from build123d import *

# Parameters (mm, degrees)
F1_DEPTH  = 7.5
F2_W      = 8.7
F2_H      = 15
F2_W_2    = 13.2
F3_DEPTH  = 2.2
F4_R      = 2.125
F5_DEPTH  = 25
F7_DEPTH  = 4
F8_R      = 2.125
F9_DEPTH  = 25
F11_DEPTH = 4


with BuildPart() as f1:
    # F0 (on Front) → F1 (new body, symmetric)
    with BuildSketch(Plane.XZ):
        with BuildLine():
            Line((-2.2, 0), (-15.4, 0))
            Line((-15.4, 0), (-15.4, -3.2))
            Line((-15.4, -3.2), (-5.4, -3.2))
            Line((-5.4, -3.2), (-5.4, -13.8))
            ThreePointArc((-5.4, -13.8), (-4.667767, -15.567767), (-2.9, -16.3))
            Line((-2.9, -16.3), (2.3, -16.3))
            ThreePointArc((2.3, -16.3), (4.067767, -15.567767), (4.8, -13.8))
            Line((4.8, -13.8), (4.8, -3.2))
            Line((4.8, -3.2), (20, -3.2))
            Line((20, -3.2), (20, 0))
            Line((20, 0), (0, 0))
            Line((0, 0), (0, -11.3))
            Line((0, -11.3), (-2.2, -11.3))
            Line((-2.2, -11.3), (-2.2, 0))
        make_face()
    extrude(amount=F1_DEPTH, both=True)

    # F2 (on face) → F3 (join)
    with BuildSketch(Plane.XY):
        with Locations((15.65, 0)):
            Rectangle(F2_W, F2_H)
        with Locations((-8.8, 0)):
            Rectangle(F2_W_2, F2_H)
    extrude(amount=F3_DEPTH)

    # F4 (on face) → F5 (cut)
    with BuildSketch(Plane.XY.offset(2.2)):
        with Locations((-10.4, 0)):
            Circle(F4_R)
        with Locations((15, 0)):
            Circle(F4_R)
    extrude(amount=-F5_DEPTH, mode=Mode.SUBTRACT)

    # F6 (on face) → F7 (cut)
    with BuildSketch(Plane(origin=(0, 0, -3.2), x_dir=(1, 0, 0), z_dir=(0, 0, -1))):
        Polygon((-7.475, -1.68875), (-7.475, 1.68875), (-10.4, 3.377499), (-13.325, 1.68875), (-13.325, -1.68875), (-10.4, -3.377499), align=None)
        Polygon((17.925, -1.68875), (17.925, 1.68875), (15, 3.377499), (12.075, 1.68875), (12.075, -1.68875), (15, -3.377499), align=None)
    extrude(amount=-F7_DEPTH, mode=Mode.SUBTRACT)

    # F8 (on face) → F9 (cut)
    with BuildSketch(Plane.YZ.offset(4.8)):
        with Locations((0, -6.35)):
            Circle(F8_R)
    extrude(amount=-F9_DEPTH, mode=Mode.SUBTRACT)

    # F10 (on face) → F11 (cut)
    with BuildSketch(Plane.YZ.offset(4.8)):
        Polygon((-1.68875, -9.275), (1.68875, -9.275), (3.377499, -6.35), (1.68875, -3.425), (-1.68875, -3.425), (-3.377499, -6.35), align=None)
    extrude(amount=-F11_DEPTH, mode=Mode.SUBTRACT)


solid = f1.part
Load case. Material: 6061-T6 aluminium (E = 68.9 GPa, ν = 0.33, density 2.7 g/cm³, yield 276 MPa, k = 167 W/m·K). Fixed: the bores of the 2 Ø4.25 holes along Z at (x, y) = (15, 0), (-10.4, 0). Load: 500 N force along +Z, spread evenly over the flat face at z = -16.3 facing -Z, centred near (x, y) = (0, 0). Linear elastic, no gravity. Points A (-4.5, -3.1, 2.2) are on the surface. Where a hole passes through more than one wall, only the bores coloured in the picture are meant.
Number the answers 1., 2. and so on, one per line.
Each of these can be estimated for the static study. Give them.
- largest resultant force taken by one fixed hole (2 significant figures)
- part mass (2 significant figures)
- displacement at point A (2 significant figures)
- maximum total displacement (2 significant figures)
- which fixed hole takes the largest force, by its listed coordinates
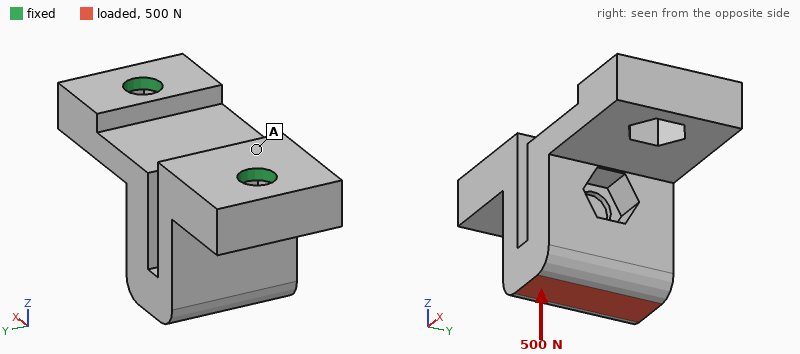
1. 330 N
2. 9.6 g
3. 5.8 µm
4. 15 µm
5. (-10.4, 0)
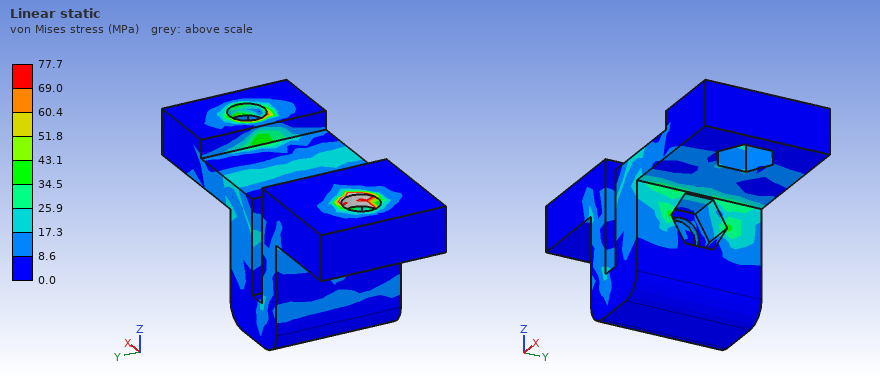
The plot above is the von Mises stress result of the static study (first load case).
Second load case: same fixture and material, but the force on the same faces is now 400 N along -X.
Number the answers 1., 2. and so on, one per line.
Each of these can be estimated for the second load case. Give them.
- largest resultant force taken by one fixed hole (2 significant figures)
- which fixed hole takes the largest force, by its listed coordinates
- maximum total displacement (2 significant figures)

1. 410 N
2. (15, 0)
3. 35 µm
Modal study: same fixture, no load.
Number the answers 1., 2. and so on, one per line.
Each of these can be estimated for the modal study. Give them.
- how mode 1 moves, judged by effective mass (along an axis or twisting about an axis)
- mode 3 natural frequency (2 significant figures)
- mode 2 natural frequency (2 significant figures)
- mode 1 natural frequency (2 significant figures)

1. along Y
2. 17 kHz
3. 12 kHz
4. 5800 Hz
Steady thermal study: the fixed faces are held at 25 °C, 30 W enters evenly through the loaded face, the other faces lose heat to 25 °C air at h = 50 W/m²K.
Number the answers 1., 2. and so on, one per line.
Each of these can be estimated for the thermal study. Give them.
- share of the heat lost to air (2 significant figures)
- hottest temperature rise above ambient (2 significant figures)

1. 8.2 %
2. 45 K
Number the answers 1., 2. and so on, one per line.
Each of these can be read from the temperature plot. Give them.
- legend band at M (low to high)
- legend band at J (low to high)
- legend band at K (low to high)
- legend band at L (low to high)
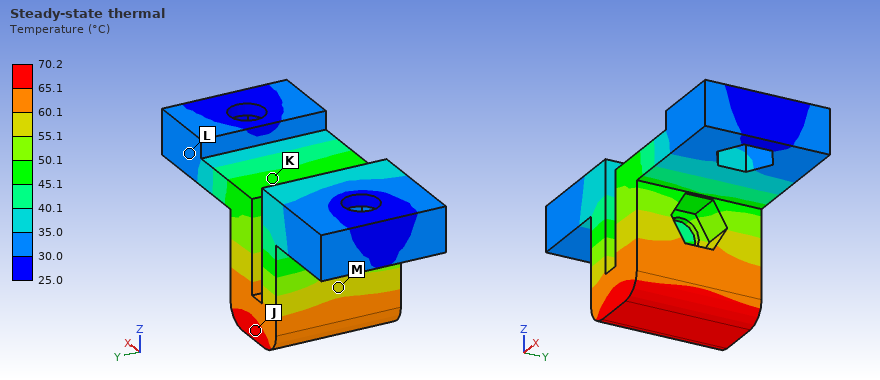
1. 55.1 to 60.1 °C
2. 65.1 to 70.2 °C
3. 45.1 to 50.1 °C
4. 30.0 to 35.0 °C
